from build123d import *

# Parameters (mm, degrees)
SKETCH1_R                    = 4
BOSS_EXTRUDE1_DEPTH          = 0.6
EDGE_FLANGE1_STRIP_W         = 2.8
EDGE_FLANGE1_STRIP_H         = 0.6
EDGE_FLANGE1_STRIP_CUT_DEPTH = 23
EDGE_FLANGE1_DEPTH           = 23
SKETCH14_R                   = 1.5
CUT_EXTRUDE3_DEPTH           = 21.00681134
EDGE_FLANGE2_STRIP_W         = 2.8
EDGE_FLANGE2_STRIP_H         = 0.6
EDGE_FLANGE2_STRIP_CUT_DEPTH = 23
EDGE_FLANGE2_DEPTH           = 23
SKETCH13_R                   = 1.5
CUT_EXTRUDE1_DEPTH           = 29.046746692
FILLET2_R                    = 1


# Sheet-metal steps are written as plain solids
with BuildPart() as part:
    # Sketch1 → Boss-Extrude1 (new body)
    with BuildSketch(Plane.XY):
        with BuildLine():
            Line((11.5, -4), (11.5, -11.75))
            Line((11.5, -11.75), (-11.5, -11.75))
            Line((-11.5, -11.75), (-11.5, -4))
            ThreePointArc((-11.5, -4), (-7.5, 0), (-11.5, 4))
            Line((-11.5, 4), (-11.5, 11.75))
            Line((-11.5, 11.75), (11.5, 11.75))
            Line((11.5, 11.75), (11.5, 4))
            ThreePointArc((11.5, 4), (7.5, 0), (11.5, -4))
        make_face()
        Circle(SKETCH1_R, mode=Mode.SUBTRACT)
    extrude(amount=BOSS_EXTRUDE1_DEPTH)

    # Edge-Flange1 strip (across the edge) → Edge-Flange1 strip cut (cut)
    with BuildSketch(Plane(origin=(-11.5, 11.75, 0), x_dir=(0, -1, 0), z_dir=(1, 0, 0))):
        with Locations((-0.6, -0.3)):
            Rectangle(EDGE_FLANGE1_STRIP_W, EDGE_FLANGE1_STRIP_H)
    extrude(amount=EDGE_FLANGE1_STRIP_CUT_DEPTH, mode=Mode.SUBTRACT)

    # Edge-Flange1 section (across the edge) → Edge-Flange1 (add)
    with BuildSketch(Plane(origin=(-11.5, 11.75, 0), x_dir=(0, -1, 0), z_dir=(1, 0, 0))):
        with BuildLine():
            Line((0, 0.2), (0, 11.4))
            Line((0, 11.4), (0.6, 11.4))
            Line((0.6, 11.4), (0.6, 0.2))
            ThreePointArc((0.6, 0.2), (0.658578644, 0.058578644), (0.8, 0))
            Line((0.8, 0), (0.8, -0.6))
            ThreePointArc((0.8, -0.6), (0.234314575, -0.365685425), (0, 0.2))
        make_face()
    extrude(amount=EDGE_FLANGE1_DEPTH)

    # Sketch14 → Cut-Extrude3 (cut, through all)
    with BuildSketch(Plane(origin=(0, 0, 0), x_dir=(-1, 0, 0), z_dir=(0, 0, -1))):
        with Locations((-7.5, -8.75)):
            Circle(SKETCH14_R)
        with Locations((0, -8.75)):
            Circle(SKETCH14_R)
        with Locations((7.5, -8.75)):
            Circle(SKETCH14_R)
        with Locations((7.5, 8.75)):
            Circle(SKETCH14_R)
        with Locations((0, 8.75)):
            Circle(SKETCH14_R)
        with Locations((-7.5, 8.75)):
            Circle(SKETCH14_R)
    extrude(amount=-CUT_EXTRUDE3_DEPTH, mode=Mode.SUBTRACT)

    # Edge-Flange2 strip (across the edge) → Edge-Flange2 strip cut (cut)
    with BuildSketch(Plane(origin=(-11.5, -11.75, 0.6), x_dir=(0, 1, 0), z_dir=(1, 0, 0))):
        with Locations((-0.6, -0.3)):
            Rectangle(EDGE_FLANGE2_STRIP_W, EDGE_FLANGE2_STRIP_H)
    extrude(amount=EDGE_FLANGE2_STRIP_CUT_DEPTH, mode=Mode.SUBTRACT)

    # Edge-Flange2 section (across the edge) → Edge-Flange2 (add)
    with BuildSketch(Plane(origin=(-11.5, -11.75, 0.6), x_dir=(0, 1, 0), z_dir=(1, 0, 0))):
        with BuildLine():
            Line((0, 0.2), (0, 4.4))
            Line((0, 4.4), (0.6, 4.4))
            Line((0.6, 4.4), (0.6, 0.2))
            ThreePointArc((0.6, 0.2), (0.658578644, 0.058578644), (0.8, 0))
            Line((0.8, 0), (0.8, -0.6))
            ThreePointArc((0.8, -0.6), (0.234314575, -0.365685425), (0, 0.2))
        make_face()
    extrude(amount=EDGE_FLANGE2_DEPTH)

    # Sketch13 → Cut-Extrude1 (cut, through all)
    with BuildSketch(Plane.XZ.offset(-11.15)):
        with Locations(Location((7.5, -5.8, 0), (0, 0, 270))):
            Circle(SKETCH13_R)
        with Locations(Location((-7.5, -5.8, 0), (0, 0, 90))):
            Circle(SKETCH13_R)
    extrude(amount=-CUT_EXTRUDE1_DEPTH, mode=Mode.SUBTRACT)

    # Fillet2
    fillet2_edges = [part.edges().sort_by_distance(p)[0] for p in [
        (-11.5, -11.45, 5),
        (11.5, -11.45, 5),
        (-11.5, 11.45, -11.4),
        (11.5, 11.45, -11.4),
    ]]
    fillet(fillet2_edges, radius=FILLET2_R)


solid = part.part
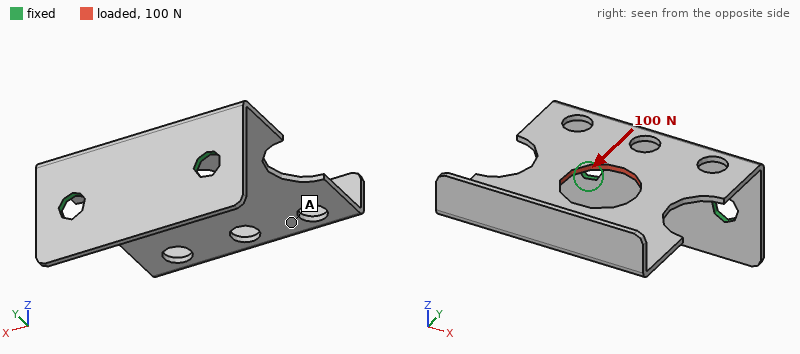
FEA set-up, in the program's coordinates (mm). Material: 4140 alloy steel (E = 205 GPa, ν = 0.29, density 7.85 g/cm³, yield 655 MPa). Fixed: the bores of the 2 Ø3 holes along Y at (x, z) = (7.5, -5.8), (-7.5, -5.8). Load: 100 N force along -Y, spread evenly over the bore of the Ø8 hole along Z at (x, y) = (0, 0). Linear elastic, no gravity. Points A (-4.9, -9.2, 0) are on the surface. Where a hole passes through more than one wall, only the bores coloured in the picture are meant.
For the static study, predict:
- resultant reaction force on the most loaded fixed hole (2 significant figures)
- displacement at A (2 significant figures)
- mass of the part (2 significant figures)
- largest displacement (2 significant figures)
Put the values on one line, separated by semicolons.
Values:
50 N; 0.33 mm; 3.5 g; 0.39 mm
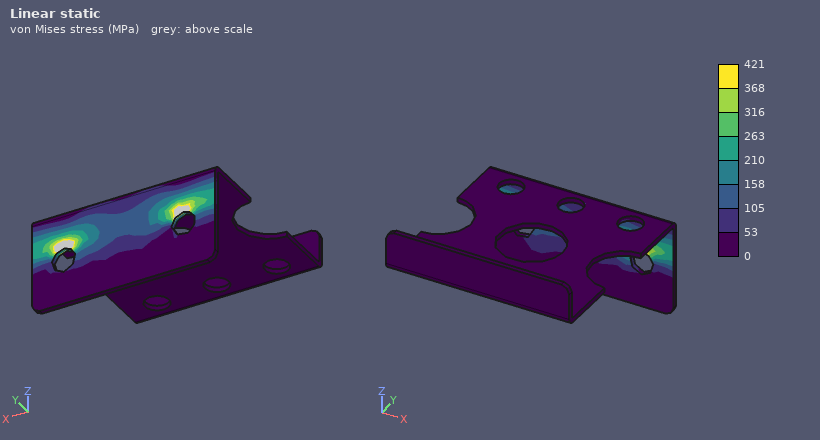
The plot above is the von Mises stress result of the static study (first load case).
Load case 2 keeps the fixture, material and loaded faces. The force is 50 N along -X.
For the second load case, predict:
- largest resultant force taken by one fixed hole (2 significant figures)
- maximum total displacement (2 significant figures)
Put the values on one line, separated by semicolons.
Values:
46 N; 0.12 mm
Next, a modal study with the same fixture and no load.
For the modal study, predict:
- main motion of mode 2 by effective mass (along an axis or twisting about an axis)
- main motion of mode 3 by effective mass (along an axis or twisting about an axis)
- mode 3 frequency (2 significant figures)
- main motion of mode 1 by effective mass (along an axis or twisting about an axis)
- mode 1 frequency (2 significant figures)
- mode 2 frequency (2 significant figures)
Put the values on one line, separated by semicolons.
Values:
twisting about Y; along X; 2300 Hz; along Z; 490 Hz; 1500 Hz
